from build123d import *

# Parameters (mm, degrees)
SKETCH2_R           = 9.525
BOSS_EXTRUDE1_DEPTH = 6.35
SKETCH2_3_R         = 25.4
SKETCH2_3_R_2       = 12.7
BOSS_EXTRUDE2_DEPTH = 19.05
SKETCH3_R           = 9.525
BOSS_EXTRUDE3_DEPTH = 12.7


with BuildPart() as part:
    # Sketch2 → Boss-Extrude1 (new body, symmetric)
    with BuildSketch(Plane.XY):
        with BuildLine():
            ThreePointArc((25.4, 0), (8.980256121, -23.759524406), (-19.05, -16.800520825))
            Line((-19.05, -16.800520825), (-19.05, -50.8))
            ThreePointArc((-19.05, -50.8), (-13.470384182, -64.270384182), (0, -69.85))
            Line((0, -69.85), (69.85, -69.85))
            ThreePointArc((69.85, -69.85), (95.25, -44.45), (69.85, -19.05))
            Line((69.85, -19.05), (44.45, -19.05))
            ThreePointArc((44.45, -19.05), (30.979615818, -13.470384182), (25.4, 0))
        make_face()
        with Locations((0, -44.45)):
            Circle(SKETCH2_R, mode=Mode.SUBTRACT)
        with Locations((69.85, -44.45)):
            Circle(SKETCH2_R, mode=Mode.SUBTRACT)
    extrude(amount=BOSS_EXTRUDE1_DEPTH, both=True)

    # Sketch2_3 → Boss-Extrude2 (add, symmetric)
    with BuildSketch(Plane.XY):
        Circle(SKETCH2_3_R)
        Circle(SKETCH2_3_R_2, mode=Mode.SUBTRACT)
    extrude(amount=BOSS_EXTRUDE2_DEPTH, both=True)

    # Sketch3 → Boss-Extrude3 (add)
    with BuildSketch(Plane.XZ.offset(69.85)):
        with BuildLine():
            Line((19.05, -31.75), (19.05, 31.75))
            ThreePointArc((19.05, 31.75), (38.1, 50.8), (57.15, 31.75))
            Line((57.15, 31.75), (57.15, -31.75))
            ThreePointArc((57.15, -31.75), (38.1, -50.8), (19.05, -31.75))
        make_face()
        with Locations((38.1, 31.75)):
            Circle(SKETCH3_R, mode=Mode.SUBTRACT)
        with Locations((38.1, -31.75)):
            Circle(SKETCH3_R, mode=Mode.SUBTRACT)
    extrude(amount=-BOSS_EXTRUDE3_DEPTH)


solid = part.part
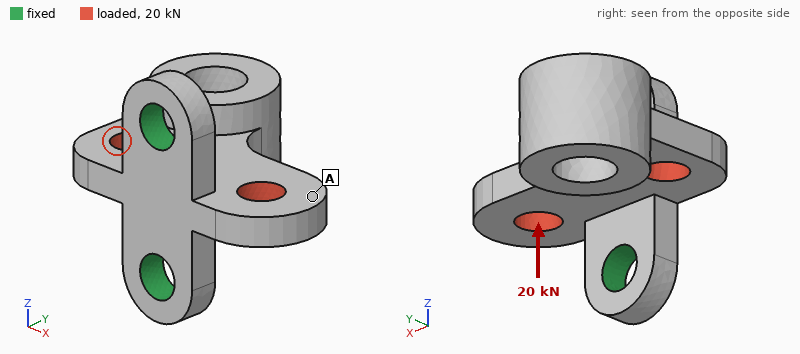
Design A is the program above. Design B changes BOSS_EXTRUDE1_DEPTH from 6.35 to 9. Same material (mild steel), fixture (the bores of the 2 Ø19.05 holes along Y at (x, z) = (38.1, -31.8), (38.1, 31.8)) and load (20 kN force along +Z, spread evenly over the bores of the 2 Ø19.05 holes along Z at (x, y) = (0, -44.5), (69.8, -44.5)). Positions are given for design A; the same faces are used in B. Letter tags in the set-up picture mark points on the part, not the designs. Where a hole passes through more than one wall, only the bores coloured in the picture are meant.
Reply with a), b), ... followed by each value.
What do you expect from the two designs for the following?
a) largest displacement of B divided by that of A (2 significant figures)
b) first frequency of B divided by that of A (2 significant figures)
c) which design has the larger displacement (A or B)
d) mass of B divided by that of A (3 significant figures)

a) 0.48
b) 1.4
c) A
d) 1.15
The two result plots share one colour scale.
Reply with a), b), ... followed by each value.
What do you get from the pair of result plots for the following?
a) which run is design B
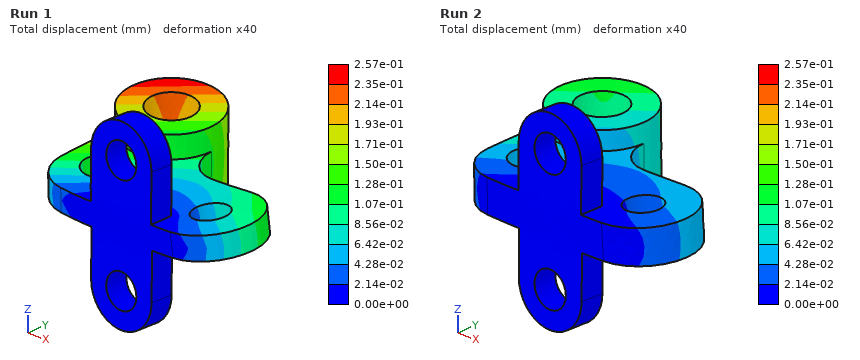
a) Run 2
